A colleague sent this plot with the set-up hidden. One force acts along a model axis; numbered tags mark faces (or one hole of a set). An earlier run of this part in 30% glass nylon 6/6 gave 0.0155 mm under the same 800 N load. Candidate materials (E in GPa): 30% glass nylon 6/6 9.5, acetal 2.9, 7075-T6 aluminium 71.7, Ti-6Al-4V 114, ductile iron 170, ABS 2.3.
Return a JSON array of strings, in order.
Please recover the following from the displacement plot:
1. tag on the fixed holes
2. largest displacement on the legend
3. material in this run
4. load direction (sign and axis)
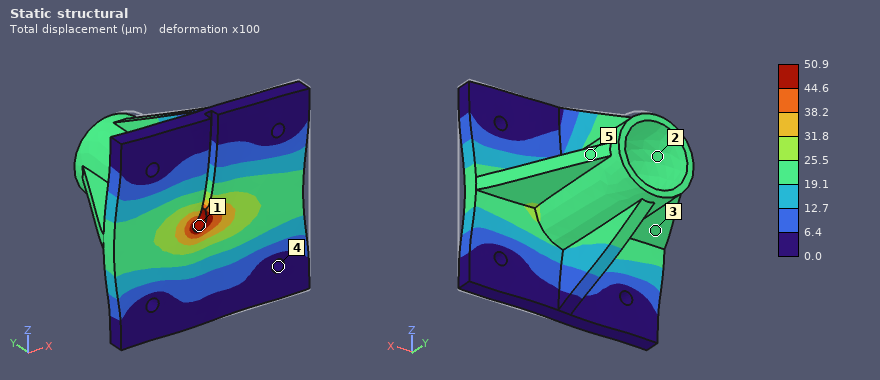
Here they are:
["4", "50.9 µm", "acetal", "-X"]
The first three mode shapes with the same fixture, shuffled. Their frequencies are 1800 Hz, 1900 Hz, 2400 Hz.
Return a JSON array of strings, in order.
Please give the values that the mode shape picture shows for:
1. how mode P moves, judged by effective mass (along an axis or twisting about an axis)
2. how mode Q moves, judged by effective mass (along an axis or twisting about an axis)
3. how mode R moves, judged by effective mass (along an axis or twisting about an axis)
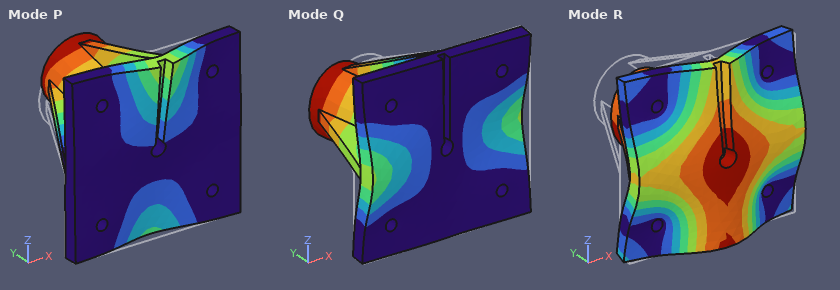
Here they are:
["along Z", "along X", "along Y"]
